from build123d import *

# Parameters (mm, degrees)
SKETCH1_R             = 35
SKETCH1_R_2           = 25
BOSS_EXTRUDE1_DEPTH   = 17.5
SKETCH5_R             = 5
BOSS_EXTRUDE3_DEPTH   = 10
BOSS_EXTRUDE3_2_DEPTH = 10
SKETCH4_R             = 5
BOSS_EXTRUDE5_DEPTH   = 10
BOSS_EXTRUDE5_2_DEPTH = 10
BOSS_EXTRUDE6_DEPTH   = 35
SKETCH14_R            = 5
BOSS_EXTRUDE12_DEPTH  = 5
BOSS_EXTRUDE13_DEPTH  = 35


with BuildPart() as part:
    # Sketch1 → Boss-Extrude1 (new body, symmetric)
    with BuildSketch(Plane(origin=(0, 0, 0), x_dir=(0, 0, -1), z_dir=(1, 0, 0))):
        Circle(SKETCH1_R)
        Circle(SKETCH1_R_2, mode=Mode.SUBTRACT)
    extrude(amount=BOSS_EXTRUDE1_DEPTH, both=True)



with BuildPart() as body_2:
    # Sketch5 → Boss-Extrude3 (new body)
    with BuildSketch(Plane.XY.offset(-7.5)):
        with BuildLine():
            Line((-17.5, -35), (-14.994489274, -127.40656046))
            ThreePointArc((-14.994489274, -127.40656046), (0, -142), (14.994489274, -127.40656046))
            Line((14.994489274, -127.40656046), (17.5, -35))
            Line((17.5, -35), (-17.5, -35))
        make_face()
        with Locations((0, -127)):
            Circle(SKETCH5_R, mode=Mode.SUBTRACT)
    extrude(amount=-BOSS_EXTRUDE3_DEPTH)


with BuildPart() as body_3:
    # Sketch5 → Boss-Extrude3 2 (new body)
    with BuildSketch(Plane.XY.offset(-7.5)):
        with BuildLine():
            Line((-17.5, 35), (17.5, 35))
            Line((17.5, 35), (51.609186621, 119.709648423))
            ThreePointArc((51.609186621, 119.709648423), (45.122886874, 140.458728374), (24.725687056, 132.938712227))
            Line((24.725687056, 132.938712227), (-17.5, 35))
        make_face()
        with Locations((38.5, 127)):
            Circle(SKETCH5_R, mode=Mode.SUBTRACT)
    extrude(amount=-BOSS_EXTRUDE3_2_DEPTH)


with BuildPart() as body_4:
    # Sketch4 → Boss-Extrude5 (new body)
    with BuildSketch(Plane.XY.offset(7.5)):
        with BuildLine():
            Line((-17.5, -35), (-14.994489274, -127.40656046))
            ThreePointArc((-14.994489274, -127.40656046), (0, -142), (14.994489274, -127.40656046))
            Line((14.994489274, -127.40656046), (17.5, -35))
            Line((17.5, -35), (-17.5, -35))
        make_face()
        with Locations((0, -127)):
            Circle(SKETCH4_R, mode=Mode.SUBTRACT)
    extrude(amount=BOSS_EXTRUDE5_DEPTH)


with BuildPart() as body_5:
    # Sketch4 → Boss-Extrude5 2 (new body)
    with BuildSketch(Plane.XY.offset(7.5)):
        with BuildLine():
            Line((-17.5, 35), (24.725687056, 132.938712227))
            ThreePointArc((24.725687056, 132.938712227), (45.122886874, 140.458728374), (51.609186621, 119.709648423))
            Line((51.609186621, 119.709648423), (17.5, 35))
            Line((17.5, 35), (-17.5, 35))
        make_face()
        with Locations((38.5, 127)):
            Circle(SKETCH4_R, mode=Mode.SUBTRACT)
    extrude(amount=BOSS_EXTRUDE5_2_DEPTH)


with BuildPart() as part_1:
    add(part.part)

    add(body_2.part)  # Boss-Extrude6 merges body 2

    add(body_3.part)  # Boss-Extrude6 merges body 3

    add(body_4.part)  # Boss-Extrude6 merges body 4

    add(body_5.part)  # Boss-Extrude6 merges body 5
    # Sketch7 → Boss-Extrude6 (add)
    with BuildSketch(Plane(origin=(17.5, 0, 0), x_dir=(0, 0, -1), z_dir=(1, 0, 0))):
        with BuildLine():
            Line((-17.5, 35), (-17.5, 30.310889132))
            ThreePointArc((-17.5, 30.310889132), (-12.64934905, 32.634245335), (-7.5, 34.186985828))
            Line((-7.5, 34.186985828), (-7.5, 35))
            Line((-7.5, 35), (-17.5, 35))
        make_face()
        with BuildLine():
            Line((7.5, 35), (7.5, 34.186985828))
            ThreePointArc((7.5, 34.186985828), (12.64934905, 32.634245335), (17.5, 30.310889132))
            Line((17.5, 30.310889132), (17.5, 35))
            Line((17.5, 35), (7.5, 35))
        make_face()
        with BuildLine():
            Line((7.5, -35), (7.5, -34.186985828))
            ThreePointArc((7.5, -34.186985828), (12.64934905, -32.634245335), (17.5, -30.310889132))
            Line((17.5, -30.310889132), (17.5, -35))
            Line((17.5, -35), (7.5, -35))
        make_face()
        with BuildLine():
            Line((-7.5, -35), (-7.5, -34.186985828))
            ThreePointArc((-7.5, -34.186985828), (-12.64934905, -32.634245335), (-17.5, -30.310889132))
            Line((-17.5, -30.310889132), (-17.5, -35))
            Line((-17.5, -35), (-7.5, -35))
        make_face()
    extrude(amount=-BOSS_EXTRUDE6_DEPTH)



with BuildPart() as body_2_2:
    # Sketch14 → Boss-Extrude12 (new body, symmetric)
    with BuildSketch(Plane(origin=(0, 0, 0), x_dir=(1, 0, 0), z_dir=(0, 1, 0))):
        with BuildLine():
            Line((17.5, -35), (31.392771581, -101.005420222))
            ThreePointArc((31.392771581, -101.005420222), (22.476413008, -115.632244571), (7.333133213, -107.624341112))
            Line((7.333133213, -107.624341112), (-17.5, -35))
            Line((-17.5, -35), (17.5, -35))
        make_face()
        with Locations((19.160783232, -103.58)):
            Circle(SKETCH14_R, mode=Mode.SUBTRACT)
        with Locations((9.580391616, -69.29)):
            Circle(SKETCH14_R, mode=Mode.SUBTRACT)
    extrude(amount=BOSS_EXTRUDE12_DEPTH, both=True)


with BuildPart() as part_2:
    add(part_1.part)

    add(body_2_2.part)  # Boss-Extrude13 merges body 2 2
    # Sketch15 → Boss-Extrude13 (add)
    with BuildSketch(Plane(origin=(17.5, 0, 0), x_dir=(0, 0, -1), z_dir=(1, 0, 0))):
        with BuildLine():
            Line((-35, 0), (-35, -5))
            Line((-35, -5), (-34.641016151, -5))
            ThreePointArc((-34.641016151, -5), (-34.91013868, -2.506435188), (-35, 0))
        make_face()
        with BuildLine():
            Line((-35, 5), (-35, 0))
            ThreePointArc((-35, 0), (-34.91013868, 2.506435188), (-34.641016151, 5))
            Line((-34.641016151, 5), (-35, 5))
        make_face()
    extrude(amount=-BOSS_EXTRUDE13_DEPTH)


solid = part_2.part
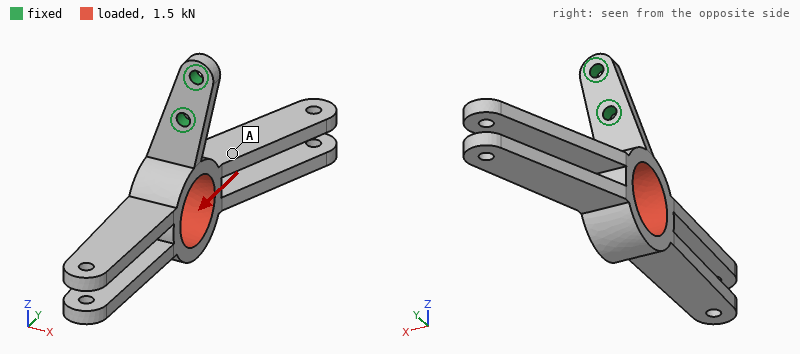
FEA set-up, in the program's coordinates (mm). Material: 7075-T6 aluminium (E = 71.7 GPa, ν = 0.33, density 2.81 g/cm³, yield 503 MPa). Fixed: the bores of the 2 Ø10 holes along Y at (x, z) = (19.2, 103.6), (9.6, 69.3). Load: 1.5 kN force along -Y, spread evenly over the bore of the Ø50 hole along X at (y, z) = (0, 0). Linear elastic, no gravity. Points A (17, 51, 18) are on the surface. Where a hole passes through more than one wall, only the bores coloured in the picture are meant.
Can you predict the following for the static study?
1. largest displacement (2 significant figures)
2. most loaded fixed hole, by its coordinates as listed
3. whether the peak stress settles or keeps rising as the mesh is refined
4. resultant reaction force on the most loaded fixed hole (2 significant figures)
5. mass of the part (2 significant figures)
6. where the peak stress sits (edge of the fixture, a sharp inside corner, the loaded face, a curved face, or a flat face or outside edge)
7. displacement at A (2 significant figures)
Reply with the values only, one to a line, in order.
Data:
2.4 mm
(9.6, 69.3)
keeps rising
1.8 kN
630 g
edge of the fixture
0.93 mm
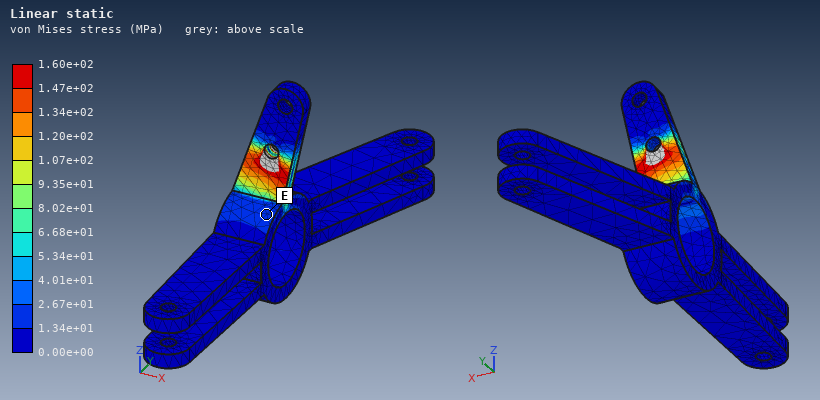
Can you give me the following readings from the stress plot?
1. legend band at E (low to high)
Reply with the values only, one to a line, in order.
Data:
1.34e+01 to 2.67e+01 MPa
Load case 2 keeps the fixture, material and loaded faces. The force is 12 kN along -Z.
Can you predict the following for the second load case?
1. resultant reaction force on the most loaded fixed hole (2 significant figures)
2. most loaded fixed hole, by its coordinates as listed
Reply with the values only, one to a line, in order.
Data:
12 kN
(9.6, 69.3)
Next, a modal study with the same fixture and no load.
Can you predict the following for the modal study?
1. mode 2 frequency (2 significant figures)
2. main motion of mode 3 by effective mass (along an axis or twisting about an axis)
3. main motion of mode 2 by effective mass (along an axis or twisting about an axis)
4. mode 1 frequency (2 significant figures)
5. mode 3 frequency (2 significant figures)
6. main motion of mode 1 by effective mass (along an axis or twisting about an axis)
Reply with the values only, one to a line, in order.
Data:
240 Hz
along X
twisting about Z
160 Hz
590 Hz
along Y
